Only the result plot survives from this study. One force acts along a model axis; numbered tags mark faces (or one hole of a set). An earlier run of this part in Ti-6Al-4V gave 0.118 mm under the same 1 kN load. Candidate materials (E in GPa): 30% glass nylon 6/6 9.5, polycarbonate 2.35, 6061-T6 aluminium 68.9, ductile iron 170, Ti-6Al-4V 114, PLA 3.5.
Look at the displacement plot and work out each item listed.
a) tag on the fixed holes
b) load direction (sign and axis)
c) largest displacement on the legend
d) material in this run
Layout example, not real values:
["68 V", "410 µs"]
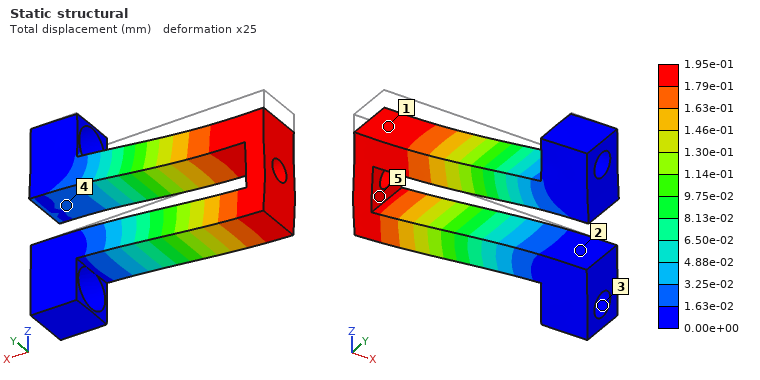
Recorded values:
["3", "-Z", "1.95e-01 mm", "6061-T6 aluminium"]
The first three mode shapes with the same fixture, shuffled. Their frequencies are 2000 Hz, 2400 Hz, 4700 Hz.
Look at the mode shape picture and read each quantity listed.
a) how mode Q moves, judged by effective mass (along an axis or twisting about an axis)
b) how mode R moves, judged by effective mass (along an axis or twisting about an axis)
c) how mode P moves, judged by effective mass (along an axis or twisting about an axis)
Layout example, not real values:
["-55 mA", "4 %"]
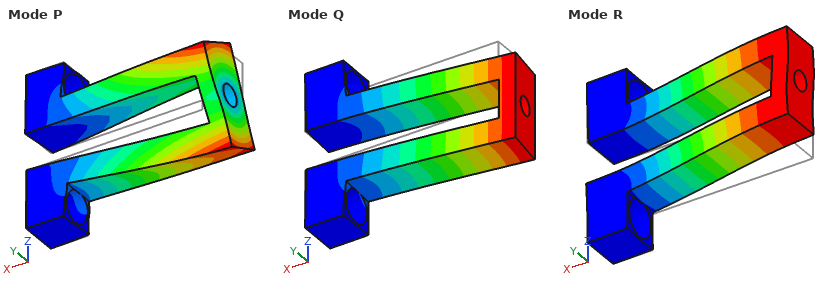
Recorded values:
["along Y", "along Z", "twisting about X"]
